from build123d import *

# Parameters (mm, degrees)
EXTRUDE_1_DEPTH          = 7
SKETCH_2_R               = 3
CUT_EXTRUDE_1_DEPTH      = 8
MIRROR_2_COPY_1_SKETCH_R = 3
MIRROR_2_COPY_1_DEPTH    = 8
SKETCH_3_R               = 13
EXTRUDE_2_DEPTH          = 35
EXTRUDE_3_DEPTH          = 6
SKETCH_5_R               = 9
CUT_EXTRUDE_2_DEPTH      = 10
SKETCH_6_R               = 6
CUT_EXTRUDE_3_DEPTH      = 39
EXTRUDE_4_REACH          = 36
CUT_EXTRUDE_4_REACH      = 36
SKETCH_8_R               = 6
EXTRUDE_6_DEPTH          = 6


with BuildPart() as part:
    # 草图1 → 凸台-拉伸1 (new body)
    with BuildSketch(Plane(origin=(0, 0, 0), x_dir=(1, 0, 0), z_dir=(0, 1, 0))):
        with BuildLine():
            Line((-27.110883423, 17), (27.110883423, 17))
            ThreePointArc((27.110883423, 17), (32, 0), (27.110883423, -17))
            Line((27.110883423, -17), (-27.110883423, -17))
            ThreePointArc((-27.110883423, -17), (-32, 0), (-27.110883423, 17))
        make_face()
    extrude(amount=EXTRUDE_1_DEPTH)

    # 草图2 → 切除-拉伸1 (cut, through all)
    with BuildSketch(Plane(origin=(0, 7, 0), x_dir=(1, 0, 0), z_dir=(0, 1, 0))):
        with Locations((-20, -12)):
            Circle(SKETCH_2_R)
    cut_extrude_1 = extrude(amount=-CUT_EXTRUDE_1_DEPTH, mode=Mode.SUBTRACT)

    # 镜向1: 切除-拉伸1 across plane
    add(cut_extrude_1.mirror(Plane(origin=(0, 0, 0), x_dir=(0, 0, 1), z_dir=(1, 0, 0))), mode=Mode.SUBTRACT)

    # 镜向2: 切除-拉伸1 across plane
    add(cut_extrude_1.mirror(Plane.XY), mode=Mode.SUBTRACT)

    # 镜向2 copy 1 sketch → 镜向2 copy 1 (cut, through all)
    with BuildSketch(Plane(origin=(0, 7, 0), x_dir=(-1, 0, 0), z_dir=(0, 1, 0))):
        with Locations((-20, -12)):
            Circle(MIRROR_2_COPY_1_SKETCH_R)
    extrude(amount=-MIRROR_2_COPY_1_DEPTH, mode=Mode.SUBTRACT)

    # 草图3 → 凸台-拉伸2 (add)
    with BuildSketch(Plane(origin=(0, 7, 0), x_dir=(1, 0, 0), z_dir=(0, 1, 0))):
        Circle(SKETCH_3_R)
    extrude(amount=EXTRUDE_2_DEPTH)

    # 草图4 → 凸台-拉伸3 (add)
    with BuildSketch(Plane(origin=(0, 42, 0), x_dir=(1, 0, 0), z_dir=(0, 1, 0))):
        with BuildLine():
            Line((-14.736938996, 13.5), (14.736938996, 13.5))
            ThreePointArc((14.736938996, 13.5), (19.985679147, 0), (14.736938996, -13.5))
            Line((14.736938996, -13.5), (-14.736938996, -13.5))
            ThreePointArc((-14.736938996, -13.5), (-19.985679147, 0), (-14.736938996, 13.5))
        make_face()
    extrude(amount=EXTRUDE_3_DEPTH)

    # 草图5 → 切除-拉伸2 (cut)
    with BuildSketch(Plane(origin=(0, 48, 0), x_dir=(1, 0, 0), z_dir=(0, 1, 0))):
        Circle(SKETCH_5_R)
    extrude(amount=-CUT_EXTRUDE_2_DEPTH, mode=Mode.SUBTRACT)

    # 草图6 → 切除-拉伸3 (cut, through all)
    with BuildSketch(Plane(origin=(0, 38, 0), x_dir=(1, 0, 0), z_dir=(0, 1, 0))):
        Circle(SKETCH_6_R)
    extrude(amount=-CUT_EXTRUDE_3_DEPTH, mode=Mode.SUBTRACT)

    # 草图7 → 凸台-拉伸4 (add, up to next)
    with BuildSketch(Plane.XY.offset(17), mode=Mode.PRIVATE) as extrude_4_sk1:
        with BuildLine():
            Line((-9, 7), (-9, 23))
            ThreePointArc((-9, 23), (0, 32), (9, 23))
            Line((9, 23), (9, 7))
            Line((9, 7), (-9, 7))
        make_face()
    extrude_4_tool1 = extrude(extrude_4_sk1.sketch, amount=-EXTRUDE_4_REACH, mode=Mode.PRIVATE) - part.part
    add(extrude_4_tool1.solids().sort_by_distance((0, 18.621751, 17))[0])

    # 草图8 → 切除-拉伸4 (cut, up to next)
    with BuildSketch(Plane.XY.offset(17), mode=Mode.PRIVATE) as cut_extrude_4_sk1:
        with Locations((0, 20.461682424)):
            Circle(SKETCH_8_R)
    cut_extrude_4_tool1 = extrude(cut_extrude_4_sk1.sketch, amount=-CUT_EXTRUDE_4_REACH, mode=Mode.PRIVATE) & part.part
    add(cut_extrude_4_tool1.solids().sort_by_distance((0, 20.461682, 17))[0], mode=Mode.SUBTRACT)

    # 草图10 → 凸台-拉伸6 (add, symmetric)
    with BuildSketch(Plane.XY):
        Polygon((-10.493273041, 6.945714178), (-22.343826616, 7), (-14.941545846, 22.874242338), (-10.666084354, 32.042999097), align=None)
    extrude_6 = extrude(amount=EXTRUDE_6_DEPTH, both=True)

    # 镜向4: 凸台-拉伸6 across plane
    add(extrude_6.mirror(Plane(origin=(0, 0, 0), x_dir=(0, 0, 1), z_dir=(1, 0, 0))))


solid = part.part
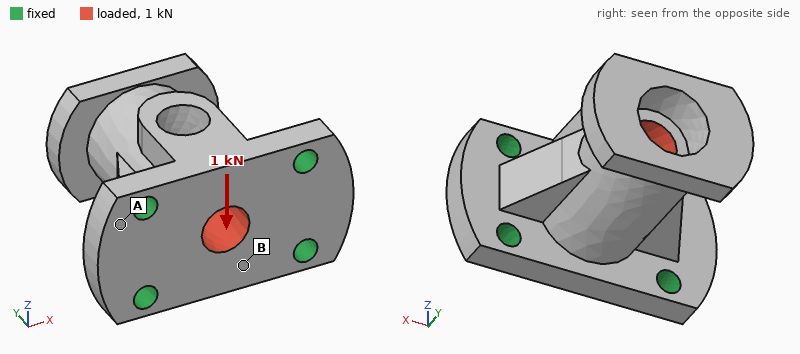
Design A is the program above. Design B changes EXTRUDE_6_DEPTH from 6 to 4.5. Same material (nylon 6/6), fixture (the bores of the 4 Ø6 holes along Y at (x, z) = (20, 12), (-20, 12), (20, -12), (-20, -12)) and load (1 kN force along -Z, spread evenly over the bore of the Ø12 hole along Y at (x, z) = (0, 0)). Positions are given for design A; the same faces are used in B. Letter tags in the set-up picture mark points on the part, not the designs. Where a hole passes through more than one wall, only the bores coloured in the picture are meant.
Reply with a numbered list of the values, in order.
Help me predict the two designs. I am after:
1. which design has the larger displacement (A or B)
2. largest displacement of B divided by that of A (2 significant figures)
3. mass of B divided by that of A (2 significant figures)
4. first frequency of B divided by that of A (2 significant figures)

1. B
2. 1.1
3. 0.98
4. 0.95
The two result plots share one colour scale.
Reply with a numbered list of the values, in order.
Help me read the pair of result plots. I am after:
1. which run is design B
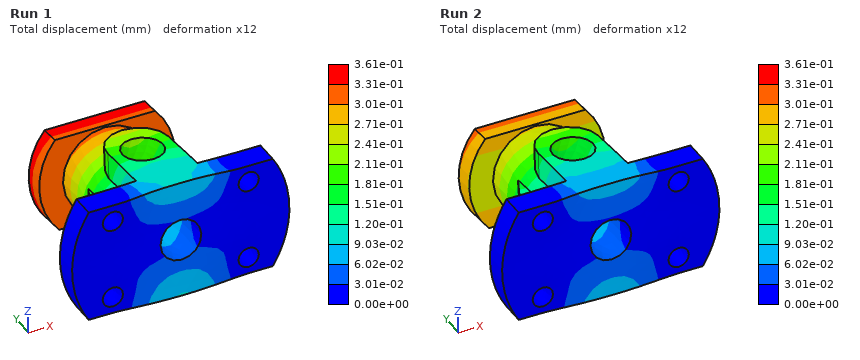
1. Run 1
